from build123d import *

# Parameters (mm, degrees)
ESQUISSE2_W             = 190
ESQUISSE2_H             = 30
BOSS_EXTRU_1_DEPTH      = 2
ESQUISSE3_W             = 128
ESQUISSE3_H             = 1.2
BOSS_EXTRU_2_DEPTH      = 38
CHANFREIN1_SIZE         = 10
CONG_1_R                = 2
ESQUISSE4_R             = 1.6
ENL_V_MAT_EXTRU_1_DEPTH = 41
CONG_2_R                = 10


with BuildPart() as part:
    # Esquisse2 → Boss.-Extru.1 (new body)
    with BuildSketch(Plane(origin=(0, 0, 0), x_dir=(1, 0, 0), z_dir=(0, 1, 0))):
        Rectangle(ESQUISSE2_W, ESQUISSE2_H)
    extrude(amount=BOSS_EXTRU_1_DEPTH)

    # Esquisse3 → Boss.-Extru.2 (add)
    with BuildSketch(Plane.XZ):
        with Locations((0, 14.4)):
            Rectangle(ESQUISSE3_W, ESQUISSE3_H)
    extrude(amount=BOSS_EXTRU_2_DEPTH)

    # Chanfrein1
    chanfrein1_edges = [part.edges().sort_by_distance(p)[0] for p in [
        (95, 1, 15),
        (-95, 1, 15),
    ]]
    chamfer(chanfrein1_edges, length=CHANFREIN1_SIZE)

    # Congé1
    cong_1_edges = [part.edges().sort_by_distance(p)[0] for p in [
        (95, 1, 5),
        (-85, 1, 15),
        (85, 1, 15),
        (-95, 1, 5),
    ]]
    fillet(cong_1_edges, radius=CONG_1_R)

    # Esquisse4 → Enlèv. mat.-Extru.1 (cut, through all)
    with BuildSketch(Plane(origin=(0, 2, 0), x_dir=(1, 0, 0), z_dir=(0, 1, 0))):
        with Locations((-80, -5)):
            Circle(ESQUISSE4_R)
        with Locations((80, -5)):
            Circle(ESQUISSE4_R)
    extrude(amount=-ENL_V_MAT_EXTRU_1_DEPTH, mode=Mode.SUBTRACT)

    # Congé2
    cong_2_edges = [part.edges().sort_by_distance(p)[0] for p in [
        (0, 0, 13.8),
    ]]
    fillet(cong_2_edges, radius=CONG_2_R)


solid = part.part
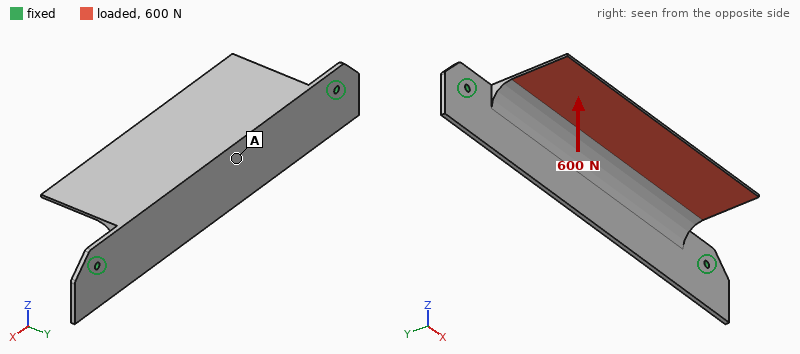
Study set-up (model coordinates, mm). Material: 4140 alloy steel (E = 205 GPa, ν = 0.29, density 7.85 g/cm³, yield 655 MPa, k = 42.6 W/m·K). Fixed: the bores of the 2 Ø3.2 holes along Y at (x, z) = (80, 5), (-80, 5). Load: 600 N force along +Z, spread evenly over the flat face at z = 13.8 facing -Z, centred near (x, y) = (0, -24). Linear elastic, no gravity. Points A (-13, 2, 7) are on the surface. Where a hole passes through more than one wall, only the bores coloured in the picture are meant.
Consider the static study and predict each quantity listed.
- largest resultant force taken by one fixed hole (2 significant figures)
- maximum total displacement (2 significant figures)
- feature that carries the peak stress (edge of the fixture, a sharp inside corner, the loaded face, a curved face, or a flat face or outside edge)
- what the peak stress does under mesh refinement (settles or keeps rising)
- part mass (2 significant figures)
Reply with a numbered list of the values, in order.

1. 310 N
2. 1.9 mm
3. edge of the fixture
4. keeps rising
5. 160 g
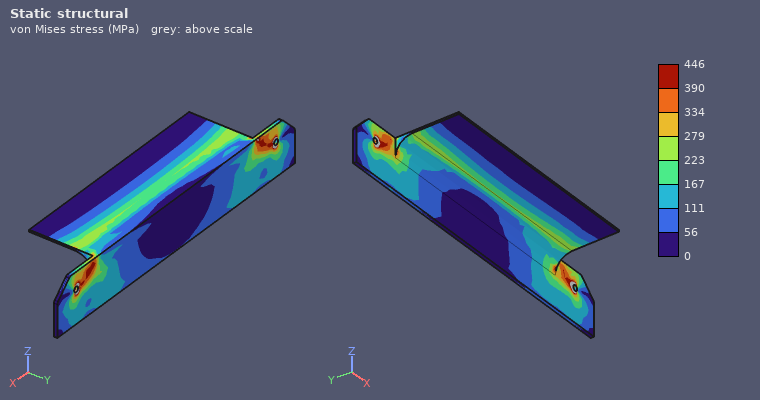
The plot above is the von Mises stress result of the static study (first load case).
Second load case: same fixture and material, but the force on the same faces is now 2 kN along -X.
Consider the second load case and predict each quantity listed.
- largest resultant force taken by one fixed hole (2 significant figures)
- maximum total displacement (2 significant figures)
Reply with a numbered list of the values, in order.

1. 1.1 kN
2. 0.23 mm
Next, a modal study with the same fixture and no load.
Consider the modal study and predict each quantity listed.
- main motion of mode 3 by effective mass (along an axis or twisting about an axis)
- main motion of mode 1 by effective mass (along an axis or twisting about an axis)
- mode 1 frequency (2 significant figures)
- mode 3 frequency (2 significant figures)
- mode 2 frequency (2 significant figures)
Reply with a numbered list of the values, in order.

1. along Y
2. along Z
3. 540 Hz
4. 1100 Hz
5. 1000 Hz
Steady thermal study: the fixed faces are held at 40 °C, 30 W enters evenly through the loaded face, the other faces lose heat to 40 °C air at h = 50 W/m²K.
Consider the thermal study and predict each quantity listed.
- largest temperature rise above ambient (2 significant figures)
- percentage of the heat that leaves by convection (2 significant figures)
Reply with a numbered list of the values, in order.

1. 78 K
2. 90 %
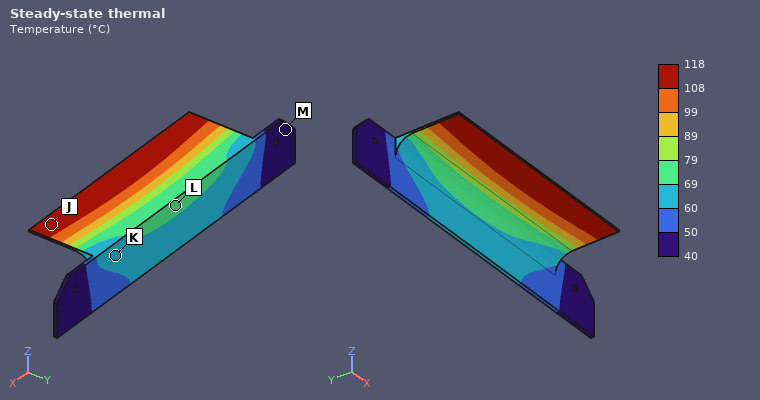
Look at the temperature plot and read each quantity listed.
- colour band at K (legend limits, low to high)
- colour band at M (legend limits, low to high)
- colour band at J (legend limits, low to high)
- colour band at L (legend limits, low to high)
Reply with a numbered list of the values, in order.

1. 60 to 69 °C
2. 40 to 50 °C
3. 108 to 118 °C
4. 69 to 79 °C
